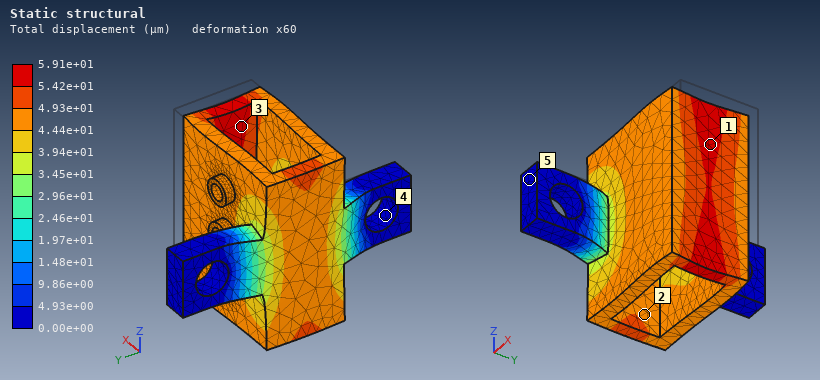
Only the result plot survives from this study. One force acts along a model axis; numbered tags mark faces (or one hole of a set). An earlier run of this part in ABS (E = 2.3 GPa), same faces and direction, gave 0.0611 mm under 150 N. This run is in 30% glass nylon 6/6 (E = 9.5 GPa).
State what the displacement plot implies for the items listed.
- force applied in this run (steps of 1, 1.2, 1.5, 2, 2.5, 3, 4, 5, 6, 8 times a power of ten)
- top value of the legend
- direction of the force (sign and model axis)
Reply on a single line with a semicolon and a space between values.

600 N; 5.91e+01 µm; -X
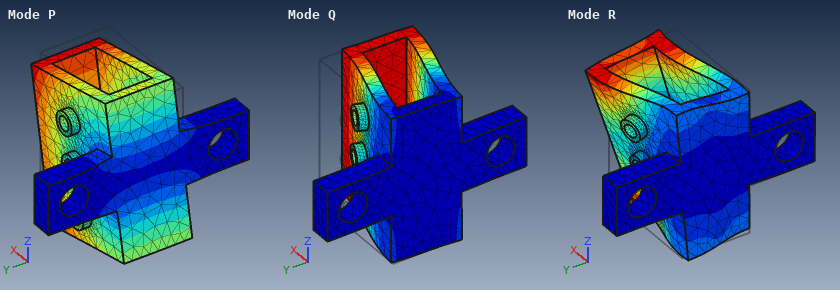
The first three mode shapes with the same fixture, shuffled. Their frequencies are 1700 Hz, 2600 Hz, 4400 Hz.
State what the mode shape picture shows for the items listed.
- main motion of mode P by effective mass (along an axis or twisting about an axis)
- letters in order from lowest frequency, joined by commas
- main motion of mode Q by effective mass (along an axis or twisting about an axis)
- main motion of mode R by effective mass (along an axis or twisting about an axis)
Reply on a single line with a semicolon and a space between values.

along Z; P, Q, R; along Y; twisting about X
